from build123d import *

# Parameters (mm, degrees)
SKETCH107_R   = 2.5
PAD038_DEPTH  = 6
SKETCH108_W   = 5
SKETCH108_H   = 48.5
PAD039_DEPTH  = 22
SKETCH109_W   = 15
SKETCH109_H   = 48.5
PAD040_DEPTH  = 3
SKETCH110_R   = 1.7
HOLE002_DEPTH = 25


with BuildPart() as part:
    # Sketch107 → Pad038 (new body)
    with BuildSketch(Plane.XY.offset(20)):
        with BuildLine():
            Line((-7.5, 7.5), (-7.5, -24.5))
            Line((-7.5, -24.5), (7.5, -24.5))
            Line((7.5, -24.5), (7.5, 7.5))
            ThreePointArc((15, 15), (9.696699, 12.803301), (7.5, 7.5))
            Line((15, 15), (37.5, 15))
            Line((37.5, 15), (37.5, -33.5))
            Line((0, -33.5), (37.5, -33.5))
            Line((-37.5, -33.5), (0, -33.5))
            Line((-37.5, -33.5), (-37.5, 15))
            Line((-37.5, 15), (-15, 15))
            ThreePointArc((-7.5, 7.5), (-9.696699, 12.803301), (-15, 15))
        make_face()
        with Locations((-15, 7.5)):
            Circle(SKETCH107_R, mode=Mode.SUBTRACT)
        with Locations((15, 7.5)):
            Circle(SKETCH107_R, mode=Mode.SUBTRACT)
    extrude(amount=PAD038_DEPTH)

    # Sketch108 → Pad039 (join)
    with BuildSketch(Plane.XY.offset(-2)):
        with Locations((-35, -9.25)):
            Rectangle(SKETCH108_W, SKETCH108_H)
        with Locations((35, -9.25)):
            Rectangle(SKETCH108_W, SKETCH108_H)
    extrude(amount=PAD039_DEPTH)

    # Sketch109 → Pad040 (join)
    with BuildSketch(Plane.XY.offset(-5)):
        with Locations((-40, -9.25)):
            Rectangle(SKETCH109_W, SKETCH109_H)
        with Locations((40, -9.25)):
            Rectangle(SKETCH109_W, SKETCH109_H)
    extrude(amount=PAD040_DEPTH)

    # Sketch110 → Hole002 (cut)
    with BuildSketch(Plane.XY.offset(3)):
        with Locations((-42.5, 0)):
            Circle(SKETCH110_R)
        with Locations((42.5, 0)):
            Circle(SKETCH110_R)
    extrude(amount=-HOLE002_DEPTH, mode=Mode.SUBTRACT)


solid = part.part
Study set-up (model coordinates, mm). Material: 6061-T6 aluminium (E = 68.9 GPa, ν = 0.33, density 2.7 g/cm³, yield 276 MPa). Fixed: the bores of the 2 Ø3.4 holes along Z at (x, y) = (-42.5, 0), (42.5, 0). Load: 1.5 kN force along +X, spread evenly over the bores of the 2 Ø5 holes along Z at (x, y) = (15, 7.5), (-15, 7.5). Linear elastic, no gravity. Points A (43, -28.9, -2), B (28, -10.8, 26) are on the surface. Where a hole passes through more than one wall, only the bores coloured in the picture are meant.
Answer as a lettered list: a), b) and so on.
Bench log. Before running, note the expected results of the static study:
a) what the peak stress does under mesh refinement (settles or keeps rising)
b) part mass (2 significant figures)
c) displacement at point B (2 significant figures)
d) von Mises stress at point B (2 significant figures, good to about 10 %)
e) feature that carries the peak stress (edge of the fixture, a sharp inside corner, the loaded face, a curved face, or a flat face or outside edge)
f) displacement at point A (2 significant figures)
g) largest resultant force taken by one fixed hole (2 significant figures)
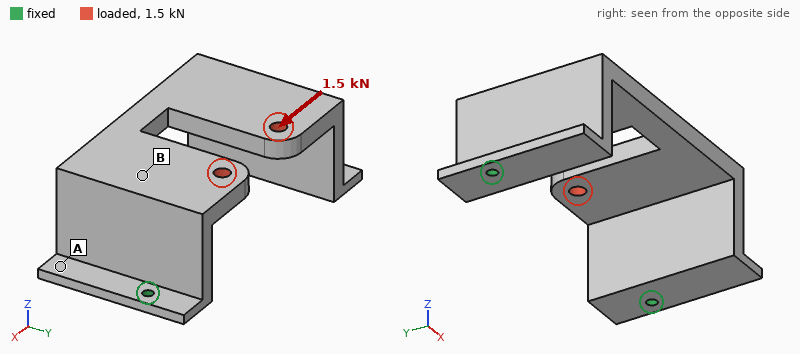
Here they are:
a) keeps rising
b) 89 g
c) 0.31 mm
d) 38 MPa
e) edge of the fixture
f) 0.21 mm
g) 830 N
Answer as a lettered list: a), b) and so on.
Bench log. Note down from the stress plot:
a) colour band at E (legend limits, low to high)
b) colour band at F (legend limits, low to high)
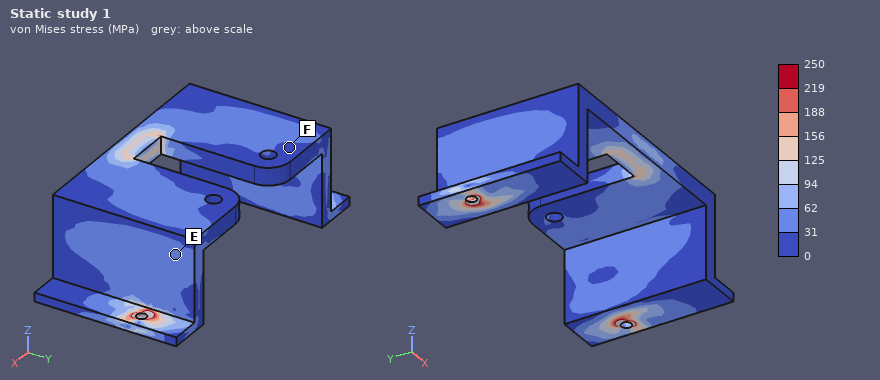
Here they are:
a) 31 to 62 MPa
b) 0 to 31 MPa
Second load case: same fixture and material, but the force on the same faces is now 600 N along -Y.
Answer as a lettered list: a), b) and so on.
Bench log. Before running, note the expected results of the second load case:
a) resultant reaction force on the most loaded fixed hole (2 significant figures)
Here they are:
a) 300 N
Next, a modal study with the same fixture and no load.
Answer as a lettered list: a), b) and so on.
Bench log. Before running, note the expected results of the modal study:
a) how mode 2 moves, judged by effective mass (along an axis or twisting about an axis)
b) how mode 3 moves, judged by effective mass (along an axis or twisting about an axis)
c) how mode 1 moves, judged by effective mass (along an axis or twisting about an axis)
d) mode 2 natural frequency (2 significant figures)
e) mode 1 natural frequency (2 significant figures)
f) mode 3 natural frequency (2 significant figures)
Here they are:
a) along X
b) along X
c) along Y
d) 1400 Hz
e) 850 Hz
f) 2000 Hz
